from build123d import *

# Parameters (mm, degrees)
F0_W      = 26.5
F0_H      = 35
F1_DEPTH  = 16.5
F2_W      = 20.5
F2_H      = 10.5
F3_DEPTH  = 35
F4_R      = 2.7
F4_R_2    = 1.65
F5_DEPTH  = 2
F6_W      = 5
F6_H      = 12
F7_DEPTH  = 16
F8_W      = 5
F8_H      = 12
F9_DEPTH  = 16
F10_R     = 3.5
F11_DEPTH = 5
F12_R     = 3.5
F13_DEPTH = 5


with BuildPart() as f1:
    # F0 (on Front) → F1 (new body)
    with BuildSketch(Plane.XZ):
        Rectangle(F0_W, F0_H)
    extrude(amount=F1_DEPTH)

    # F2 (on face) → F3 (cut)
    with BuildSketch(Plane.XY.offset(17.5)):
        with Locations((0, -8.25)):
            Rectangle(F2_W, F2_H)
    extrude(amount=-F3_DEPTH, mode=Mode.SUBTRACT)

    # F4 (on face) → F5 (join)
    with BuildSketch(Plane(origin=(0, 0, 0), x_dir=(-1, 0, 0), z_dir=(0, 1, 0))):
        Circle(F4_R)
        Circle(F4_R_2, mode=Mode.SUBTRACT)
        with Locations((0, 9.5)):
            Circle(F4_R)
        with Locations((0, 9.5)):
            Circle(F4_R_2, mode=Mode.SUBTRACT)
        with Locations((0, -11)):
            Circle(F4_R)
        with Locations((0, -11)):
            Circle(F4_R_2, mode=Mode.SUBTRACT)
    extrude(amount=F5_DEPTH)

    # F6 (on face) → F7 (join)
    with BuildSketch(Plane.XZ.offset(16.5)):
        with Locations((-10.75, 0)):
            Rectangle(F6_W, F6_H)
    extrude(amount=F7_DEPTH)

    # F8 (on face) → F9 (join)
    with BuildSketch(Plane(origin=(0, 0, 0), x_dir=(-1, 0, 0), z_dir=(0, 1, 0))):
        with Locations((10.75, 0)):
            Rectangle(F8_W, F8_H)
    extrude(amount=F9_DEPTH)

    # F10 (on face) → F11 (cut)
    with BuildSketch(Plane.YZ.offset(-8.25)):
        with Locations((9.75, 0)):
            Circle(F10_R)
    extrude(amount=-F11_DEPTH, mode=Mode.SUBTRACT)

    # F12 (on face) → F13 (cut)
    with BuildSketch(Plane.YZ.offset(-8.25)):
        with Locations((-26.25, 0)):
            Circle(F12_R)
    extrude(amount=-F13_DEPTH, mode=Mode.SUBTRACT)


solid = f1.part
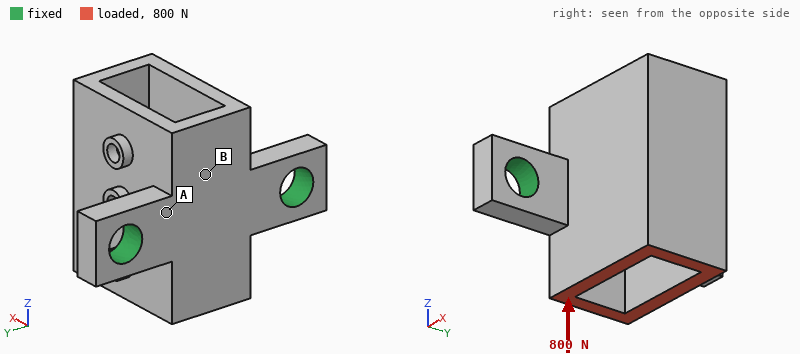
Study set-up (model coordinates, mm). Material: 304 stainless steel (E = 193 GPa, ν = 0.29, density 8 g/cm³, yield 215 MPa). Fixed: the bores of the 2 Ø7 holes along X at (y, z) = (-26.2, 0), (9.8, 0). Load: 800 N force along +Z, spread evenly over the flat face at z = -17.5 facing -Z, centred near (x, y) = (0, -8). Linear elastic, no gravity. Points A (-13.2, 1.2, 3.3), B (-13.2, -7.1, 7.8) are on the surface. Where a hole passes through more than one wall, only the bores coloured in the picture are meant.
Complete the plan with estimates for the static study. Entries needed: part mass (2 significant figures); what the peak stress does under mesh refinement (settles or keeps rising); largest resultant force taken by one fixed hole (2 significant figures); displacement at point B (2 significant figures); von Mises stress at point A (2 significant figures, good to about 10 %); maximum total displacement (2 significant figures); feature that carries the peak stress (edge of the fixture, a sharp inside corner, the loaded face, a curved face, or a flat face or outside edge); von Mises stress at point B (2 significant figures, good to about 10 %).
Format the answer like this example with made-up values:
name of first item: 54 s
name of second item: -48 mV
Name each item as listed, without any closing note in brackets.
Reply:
part mass: 75 g
what the peak stress does under mesh refinement: keeps rising
largest resultant force taken by one fixed hole: 400 N
displacement at point B: 8.7 µm
von Mises stress at point A: 48 MPa
maximum total displacement: 35 µm
feature that carries the peak stress: edge of the fixture
von Mises stress at point B: 11 MPa
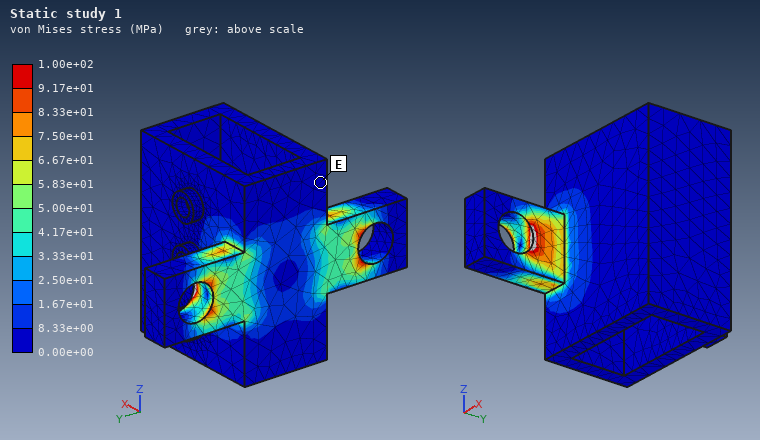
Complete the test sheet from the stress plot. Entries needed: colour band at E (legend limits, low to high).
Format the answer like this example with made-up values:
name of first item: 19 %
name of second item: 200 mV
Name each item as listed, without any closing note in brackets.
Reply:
colour band at E: 0.00e+00 to 8.33e+00 MPa
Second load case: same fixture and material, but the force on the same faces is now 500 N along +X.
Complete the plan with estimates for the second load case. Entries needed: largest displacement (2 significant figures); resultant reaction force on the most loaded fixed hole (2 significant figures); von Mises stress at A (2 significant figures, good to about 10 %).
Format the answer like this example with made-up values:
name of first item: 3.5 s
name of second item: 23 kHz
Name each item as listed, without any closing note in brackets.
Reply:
largest displacement: 36 µm
resultant reaction force on the most loaded fixed hole: 260 N
von Mises stress at A: 60 MPa
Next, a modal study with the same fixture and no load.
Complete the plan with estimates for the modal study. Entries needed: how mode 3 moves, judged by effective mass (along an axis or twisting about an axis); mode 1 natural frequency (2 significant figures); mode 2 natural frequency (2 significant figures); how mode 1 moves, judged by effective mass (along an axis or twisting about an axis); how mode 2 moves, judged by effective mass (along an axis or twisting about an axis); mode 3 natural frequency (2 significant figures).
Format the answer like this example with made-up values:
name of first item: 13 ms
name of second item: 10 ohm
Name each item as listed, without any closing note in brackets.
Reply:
how mode 3 moves, judged by effective mass: twisting about X
mode 1 natural frequency: 3200 Hz
mode 2 natural frequency: 4800 Hz
how mode 1 moves, judged by effective mass: along Z
how mode 2 moves, judged by effective mass: along Y
mode 3 natural frequency: 8300 Hz
